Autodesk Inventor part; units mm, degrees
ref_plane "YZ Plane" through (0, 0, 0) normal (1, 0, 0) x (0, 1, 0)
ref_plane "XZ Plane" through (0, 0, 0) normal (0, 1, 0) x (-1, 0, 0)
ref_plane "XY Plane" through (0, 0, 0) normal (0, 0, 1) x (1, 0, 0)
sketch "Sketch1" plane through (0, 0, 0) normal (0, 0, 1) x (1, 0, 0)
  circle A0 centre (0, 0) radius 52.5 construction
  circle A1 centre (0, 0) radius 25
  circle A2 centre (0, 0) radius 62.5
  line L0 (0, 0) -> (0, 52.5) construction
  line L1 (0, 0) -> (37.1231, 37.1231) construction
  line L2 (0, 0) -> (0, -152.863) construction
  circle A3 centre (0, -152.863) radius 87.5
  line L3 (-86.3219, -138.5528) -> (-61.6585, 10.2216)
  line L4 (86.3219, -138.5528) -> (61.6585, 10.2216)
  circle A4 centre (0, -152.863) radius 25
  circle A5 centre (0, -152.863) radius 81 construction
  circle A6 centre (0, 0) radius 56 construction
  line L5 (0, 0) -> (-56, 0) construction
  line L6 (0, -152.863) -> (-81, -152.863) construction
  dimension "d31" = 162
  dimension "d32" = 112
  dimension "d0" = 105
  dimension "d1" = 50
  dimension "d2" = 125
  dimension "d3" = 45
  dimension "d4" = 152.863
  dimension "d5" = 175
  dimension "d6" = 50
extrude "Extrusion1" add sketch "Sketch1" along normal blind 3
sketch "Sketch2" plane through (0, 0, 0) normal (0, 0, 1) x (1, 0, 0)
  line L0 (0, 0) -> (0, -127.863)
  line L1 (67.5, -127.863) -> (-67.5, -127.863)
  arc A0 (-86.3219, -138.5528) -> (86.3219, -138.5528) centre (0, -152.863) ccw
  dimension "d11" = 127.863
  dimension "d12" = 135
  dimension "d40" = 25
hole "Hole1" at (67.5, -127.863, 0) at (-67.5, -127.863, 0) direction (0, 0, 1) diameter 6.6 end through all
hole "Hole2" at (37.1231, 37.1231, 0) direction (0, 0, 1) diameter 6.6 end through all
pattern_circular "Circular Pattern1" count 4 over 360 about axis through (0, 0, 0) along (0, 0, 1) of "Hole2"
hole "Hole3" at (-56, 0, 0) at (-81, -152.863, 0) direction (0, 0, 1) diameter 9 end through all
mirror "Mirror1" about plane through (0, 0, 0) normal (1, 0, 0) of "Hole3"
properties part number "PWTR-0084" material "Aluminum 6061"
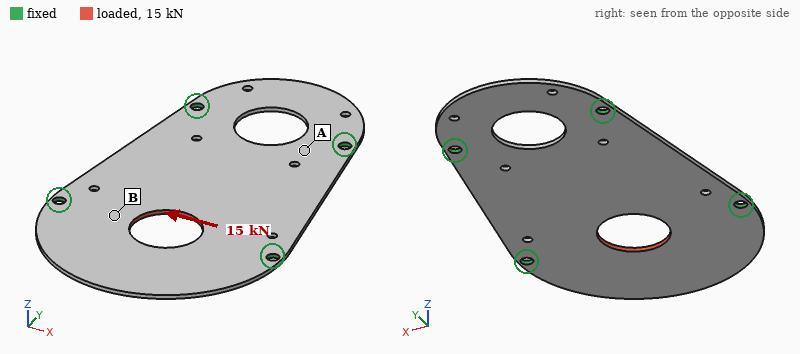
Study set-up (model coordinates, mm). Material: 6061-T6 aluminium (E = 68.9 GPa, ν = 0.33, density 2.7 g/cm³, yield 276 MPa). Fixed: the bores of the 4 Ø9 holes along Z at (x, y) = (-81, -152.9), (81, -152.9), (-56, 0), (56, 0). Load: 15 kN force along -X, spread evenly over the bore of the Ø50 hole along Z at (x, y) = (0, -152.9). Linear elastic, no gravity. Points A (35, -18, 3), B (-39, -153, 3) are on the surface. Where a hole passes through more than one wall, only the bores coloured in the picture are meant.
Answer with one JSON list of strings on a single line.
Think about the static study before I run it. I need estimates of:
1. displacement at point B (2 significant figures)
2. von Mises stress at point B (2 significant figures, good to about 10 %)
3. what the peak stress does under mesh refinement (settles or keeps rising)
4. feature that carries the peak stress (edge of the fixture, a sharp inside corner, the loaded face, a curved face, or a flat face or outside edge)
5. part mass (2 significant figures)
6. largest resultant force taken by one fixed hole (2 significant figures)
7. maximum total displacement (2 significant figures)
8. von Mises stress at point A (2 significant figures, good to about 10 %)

["38 µm", "43 MPa", "keeps rising", "edge of the fixture", "300 g", "6.7 kN", "61 µm", "14 MPa"]
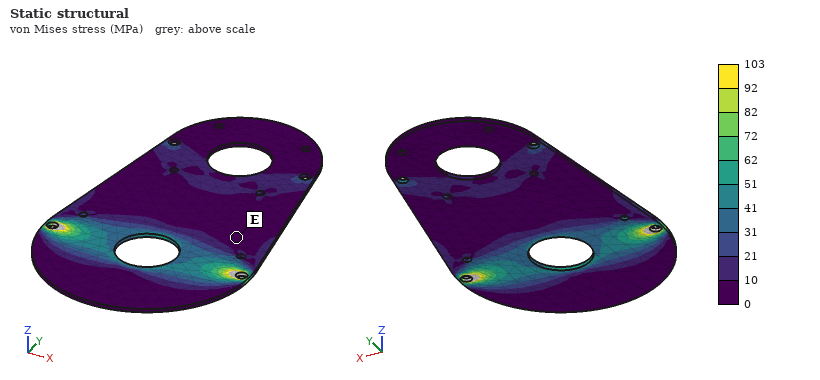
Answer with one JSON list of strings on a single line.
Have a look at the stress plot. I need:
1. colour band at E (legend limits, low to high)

["0 to 10 MPa"]
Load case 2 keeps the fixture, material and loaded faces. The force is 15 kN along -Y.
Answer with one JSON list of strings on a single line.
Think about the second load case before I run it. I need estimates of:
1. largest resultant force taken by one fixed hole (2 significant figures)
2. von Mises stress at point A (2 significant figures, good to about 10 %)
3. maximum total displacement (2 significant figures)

["4.7 kN", "18 MPa", "69 µm"]
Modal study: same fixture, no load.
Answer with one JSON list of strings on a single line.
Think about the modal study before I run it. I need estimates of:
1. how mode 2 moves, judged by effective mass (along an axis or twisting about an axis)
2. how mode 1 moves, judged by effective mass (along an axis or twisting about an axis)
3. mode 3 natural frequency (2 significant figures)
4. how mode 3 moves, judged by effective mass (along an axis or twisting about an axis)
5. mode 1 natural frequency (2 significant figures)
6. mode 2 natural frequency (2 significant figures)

["along Z", "along Z", "580 Hz", "along Z", "280 Hz", "480 Hz"]
